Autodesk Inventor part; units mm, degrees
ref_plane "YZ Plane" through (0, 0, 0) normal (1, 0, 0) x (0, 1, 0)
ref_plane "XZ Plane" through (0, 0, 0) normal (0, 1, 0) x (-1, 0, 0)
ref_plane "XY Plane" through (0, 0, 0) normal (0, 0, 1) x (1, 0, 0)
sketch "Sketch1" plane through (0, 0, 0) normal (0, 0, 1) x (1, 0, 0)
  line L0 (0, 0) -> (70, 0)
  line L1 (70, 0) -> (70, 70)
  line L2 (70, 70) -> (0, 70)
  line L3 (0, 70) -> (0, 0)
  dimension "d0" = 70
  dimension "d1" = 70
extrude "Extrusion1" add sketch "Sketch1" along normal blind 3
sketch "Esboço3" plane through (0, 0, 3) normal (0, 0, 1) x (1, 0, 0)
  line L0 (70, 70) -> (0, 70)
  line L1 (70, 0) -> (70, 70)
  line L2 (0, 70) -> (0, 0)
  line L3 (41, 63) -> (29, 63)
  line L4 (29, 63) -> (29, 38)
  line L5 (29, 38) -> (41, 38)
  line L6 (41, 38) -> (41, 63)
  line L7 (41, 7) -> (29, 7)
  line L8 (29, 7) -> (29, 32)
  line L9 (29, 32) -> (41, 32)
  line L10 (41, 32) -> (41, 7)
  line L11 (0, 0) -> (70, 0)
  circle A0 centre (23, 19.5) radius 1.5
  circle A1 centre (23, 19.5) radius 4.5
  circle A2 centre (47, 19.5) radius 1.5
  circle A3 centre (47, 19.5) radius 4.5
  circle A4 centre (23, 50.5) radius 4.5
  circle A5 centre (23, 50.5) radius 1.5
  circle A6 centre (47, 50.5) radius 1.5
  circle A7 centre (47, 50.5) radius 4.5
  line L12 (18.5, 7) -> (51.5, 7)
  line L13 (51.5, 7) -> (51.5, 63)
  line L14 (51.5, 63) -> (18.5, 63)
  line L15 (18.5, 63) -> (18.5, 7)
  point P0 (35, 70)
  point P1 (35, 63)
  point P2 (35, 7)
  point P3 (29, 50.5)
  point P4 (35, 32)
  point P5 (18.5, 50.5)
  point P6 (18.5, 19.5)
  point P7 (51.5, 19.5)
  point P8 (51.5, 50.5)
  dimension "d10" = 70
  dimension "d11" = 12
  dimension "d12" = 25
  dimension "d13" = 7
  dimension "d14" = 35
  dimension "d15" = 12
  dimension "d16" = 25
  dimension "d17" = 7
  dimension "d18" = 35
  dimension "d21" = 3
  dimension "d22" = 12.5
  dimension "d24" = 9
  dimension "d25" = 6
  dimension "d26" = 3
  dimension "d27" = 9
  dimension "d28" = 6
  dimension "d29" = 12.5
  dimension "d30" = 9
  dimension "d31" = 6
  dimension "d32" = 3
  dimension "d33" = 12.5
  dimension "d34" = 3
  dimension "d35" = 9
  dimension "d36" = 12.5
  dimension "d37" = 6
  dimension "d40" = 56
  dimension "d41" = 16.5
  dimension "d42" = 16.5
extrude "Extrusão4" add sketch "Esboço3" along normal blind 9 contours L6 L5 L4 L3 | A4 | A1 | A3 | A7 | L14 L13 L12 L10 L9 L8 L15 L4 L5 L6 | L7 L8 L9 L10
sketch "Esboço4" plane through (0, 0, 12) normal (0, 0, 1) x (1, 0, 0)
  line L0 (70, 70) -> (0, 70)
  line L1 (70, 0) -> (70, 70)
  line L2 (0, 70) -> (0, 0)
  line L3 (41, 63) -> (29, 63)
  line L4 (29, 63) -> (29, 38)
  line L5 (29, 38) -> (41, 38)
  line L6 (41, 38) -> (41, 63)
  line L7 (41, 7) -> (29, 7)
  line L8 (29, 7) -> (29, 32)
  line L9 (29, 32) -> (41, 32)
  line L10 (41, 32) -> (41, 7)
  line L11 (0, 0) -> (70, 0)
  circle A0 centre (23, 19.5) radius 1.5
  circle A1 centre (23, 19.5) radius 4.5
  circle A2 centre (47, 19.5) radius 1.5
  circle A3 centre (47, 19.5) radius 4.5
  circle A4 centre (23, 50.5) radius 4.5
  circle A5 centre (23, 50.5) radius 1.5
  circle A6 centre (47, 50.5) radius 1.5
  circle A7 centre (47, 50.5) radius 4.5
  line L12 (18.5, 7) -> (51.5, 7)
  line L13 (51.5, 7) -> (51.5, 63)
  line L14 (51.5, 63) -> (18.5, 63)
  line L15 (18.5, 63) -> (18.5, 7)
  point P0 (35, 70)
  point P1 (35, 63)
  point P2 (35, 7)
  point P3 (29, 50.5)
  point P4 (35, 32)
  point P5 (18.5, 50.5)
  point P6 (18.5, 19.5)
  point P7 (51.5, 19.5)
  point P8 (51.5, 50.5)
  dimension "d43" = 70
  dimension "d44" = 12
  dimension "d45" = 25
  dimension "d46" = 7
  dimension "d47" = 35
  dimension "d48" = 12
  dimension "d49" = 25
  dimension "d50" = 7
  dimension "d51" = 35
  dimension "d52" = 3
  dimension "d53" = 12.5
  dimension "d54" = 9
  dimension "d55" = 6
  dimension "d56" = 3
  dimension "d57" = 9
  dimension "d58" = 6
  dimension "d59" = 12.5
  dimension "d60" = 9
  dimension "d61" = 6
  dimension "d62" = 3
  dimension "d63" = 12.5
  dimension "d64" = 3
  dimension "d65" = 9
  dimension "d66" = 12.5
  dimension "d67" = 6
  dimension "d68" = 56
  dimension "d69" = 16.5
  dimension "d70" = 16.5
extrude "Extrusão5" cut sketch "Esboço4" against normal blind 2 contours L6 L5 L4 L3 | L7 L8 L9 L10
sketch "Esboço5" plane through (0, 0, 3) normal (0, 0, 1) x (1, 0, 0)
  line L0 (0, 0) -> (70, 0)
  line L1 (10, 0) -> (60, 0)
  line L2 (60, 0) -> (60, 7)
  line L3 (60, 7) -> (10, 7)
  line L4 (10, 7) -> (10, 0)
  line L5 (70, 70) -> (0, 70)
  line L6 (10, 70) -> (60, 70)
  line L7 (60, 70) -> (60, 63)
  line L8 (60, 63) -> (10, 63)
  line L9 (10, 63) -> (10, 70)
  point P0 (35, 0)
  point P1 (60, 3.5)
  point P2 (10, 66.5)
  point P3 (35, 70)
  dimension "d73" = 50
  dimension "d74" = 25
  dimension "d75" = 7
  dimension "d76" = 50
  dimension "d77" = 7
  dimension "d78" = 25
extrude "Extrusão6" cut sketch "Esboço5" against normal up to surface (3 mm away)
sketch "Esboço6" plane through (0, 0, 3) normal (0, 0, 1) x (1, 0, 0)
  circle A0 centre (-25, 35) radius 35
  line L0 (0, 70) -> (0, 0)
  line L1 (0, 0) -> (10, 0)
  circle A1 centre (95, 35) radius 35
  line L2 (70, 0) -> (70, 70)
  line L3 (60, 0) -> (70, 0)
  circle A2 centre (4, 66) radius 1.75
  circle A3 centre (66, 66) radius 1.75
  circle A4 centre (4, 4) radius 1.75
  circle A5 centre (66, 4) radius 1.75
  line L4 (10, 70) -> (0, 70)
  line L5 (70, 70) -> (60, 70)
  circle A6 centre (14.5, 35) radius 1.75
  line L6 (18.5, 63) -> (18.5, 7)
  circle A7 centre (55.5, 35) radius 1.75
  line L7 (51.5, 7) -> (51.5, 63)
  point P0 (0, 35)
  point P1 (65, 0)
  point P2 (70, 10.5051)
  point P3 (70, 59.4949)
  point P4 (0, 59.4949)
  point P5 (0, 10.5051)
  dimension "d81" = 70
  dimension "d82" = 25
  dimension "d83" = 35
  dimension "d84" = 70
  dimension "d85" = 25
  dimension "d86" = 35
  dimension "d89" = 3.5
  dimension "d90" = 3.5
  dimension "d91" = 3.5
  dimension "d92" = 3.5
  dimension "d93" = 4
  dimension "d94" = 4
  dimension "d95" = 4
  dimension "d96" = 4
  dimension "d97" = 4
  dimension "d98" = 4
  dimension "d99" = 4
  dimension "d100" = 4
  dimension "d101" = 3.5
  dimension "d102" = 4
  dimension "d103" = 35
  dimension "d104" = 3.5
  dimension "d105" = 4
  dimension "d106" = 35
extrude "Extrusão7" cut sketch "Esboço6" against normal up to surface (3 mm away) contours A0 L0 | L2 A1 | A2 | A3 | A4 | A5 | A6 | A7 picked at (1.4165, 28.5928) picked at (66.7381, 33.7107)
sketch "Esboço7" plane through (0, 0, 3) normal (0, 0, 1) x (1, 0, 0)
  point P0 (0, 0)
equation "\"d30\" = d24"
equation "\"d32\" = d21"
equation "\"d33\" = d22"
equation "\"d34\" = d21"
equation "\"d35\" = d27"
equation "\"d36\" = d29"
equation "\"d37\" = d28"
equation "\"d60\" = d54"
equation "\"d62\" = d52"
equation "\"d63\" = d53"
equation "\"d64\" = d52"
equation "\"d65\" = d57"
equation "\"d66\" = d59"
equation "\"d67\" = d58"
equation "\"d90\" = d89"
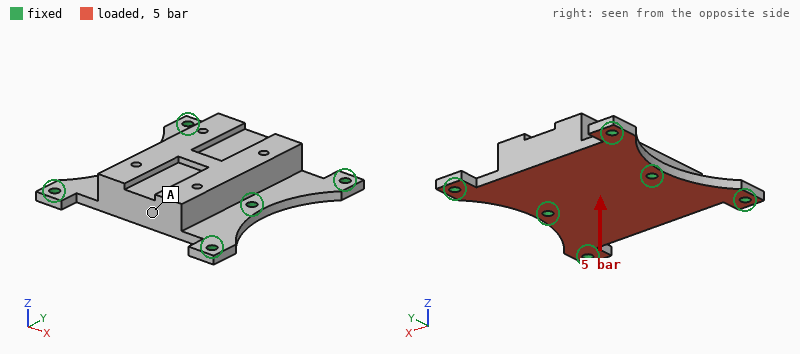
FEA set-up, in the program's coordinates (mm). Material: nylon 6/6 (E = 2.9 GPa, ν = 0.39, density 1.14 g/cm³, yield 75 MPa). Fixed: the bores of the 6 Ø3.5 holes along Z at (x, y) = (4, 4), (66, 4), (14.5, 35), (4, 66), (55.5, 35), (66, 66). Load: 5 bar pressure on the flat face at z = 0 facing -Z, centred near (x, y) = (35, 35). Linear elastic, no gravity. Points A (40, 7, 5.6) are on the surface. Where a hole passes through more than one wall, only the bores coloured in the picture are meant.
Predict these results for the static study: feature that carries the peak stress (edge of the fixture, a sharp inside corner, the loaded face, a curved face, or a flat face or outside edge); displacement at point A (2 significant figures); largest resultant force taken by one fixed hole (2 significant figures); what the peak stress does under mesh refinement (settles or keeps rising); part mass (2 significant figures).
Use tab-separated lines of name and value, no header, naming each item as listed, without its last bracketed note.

feature that carries the peak stress	edge of the fixture
displacement at point A	0.30 mm
largest resultant force taken by one fixed hole	720 N
what the peak stress does under mesh refinement	keeps rising
part mass	29 g
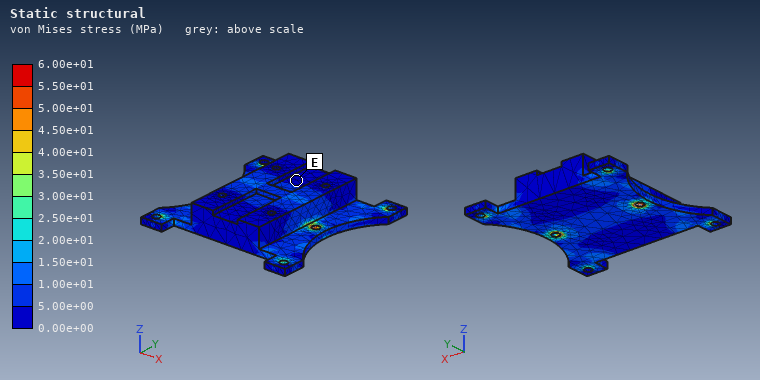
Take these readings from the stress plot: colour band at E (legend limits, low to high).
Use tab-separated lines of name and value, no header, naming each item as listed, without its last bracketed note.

colour band at E	0.00e+00 to 5.00e+00 MPa
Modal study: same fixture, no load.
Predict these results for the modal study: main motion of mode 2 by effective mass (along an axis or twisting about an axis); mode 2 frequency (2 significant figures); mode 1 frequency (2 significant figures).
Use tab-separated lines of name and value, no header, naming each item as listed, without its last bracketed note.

main motion of mode 2 by effective mass	along Z
mode 2 frequency	2300 Hz
mode 1 frequency	1300 Hz
